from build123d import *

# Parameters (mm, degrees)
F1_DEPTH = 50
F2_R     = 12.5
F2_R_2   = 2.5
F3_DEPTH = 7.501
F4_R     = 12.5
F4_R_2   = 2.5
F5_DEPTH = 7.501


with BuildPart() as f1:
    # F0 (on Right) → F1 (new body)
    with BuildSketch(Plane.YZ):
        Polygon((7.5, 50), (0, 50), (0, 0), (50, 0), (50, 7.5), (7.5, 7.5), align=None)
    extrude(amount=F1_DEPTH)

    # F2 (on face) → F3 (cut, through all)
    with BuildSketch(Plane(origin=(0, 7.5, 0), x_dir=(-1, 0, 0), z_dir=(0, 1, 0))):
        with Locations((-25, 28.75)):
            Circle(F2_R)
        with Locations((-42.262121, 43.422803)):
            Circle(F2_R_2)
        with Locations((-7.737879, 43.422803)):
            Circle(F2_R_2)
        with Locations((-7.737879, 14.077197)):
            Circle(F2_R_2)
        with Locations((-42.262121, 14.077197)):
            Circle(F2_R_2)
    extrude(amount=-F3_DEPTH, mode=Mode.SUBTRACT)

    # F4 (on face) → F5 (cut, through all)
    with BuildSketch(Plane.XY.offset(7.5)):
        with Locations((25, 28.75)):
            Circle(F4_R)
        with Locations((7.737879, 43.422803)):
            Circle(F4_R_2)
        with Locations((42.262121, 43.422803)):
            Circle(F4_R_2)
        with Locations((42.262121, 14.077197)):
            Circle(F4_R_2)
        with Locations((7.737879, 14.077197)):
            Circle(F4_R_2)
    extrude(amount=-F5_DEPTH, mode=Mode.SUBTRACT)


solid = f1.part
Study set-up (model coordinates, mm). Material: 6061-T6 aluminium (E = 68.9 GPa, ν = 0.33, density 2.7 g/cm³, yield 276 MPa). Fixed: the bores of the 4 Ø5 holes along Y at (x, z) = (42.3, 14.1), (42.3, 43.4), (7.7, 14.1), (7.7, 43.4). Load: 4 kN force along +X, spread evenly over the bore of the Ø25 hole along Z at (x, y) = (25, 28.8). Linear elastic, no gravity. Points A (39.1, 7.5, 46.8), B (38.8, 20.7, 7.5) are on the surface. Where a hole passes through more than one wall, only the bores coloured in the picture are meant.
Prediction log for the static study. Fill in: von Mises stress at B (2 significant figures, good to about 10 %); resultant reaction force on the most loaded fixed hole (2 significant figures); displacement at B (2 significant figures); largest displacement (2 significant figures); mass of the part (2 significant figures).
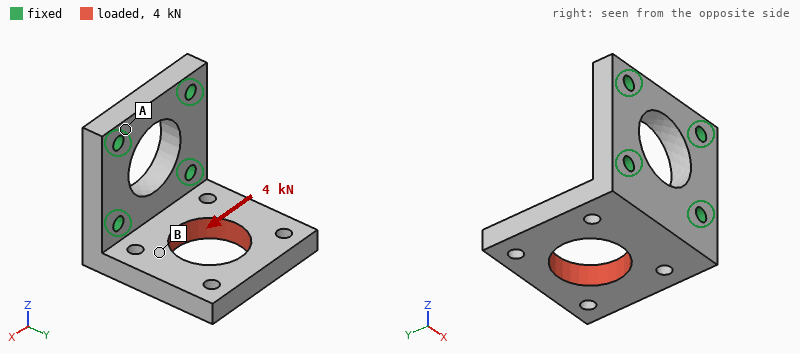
31 MPa
3.4 kN
0.042 mm
0.12 mm
71 g
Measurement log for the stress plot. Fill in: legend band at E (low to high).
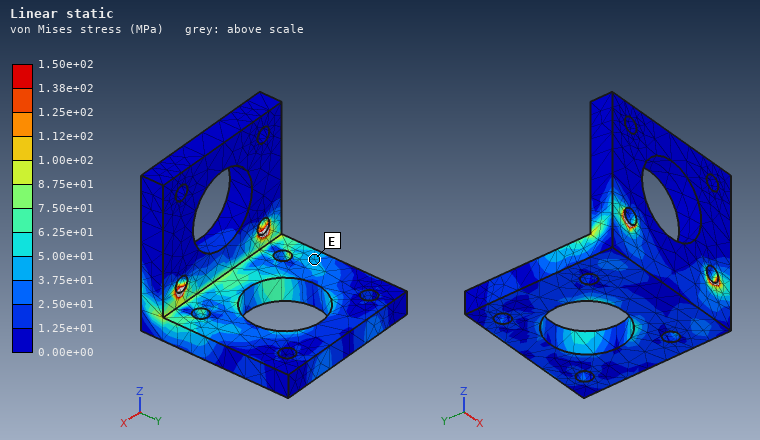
3.75e+01 to 5.00e+01 MPa
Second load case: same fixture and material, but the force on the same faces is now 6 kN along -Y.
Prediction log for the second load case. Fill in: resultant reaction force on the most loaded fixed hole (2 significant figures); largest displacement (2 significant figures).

3.1 kN
0.17 mm
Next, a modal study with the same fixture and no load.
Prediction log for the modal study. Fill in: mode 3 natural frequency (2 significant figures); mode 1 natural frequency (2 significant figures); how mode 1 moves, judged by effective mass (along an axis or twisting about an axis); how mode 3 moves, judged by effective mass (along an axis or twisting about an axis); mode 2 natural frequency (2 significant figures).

6500 Hz
2100 Hz
along Z
along X
4600 Hz
